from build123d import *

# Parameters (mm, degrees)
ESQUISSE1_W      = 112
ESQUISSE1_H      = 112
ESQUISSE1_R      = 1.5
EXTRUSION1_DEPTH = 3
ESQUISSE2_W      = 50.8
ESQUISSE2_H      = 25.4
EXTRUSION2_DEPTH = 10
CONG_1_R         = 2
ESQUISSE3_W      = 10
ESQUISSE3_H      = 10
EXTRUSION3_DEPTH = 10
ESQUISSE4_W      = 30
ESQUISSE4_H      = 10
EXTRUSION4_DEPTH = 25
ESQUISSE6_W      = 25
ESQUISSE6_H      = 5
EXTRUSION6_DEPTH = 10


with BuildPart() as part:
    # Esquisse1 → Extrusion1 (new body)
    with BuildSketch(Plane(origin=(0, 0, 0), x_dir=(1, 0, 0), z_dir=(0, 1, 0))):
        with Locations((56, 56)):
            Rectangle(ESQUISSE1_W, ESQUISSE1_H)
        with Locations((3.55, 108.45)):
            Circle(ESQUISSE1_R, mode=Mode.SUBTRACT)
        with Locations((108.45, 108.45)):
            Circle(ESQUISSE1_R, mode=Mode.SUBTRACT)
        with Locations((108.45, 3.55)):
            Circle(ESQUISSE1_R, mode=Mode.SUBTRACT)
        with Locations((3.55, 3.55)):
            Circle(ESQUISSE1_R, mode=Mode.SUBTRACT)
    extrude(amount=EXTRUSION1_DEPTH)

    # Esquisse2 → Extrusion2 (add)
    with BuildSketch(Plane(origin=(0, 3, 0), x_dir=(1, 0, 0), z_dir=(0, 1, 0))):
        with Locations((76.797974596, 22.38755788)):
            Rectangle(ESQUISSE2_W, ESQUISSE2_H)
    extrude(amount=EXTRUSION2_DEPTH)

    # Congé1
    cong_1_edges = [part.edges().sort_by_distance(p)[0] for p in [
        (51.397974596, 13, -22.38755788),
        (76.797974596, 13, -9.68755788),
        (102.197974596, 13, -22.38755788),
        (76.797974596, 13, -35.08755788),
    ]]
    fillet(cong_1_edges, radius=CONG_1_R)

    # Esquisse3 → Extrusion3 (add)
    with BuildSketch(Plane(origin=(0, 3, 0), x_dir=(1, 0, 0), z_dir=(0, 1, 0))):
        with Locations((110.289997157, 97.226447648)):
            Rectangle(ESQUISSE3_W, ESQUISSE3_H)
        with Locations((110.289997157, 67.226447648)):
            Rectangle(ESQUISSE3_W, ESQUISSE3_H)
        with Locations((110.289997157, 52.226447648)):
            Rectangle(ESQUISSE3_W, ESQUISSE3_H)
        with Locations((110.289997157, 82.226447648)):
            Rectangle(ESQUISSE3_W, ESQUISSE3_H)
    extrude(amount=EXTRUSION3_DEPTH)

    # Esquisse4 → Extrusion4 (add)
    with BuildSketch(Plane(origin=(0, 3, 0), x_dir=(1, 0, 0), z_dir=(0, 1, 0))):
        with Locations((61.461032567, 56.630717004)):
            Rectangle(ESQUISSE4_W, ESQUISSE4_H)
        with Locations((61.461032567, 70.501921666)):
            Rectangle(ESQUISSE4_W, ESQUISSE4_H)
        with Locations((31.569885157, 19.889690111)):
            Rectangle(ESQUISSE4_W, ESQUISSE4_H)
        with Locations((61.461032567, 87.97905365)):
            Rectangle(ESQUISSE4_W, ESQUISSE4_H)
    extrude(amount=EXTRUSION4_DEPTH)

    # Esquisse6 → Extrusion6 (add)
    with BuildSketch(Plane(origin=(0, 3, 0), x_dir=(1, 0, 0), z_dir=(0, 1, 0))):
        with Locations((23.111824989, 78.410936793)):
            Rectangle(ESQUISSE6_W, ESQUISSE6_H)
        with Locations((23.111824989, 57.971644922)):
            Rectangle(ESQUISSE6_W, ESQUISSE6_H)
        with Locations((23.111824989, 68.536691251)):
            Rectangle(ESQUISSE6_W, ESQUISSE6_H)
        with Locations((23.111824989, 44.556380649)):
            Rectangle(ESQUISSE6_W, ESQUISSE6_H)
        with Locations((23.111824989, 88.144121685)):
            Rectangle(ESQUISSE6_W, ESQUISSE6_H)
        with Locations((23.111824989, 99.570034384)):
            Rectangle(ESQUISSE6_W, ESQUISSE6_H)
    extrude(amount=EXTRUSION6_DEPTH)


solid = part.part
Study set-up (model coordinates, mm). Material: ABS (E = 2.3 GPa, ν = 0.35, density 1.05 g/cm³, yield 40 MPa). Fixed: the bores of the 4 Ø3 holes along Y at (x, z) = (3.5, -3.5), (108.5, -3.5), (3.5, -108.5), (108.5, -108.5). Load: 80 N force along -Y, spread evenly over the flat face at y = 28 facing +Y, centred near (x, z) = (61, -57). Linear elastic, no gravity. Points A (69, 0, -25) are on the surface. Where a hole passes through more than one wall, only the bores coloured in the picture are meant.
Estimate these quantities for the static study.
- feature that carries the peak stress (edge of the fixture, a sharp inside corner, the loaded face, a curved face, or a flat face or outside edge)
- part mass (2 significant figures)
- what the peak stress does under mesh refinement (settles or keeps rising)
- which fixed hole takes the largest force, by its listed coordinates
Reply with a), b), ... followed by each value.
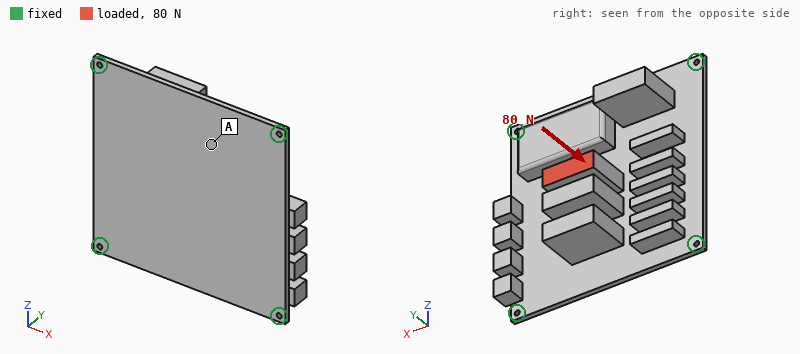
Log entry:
a) edge of the fixture
b) 96 g
c) keeps rising
d) (108.5, -3.5)
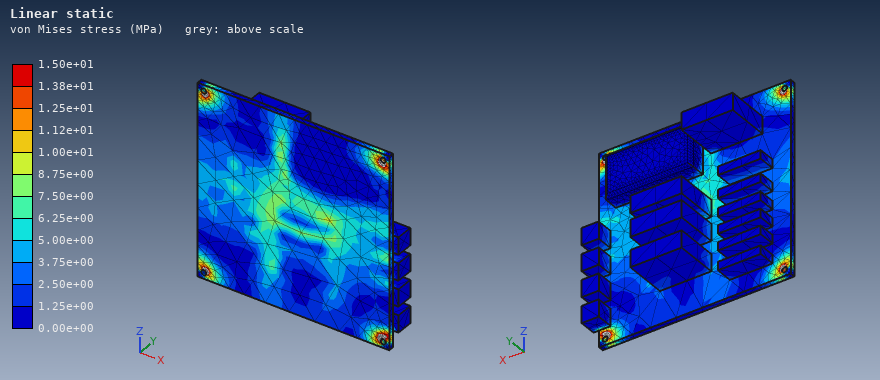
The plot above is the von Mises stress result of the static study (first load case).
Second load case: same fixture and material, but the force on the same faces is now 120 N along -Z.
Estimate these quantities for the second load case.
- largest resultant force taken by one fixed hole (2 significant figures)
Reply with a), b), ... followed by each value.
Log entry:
a) 44 N
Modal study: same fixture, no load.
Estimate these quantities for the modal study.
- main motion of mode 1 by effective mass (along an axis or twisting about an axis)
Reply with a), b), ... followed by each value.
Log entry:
a) along Y
